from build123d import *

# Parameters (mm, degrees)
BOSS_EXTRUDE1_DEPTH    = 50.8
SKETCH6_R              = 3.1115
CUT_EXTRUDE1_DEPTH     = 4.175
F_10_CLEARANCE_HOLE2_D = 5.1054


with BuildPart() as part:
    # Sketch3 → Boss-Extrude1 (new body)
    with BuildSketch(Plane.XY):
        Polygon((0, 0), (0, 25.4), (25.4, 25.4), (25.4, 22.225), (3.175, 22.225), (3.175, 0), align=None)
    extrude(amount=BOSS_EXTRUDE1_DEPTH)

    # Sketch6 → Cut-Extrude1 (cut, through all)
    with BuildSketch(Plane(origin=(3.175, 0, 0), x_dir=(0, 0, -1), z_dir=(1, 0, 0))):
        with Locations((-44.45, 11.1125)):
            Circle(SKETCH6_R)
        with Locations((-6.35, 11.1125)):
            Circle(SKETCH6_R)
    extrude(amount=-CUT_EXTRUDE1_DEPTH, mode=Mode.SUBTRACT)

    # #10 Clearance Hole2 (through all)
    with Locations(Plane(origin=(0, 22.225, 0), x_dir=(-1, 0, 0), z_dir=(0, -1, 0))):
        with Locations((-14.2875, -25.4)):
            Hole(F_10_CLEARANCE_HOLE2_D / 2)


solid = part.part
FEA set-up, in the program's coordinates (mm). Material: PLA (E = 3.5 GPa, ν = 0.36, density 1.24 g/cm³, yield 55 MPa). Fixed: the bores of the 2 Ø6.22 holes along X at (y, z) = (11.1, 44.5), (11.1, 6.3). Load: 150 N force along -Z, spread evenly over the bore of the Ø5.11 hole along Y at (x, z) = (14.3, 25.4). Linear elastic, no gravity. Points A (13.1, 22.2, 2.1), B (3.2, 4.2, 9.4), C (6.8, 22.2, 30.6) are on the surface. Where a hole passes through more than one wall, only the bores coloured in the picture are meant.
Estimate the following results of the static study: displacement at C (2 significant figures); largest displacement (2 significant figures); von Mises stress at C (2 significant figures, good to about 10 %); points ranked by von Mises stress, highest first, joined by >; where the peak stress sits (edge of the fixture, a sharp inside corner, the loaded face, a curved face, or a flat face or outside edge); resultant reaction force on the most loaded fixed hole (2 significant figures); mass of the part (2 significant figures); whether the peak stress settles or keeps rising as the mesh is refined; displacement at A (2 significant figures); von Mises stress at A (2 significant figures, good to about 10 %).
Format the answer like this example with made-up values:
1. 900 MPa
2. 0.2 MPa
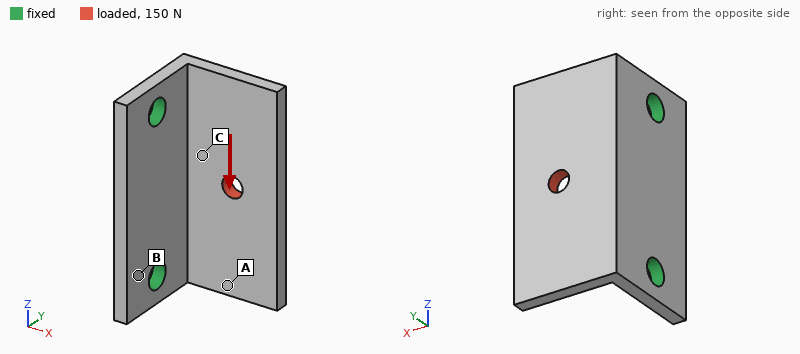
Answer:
1. 0.045 mm
2. 0.22 mm
3. 4.5 MPa
4. C > A > B
5. edge of the fixture
6. 99 N
7. 9.2 g
8. keeps rising
9. 0.14 mm
10. 2.3 MPa
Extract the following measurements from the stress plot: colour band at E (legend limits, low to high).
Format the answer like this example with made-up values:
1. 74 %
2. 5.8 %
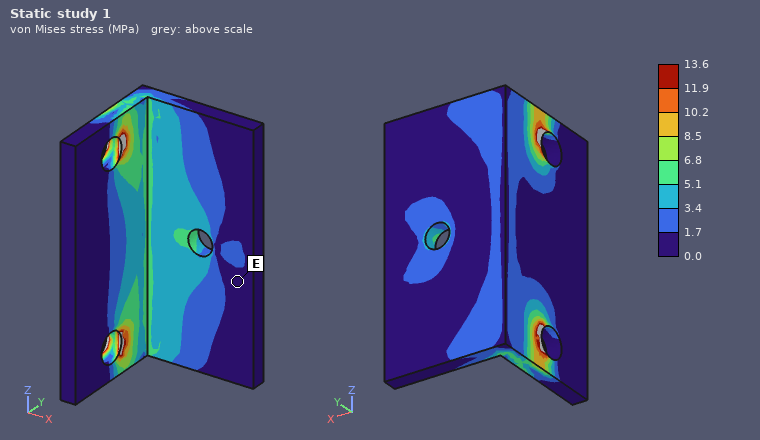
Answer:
1. 0.0 to 1.7 MPa
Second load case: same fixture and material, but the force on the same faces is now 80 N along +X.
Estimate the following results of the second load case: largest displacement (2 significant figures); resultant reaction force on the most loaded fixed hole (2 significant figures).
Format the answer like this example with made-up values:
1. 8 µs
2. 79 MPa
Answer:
1. 0.30 mm
2. 41 N
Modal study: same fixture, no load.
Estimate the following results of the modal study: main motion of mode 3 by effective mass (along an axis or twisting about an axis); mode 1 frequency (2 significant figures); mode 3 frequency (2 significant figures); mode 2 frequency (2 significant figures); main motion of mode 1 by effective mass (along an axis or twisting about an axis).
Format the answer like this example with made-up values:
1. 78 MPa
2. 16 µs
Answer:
1. along X
2. 880 Hz
3. 2700 Hz
4. 1600 Hz
5. along Y
